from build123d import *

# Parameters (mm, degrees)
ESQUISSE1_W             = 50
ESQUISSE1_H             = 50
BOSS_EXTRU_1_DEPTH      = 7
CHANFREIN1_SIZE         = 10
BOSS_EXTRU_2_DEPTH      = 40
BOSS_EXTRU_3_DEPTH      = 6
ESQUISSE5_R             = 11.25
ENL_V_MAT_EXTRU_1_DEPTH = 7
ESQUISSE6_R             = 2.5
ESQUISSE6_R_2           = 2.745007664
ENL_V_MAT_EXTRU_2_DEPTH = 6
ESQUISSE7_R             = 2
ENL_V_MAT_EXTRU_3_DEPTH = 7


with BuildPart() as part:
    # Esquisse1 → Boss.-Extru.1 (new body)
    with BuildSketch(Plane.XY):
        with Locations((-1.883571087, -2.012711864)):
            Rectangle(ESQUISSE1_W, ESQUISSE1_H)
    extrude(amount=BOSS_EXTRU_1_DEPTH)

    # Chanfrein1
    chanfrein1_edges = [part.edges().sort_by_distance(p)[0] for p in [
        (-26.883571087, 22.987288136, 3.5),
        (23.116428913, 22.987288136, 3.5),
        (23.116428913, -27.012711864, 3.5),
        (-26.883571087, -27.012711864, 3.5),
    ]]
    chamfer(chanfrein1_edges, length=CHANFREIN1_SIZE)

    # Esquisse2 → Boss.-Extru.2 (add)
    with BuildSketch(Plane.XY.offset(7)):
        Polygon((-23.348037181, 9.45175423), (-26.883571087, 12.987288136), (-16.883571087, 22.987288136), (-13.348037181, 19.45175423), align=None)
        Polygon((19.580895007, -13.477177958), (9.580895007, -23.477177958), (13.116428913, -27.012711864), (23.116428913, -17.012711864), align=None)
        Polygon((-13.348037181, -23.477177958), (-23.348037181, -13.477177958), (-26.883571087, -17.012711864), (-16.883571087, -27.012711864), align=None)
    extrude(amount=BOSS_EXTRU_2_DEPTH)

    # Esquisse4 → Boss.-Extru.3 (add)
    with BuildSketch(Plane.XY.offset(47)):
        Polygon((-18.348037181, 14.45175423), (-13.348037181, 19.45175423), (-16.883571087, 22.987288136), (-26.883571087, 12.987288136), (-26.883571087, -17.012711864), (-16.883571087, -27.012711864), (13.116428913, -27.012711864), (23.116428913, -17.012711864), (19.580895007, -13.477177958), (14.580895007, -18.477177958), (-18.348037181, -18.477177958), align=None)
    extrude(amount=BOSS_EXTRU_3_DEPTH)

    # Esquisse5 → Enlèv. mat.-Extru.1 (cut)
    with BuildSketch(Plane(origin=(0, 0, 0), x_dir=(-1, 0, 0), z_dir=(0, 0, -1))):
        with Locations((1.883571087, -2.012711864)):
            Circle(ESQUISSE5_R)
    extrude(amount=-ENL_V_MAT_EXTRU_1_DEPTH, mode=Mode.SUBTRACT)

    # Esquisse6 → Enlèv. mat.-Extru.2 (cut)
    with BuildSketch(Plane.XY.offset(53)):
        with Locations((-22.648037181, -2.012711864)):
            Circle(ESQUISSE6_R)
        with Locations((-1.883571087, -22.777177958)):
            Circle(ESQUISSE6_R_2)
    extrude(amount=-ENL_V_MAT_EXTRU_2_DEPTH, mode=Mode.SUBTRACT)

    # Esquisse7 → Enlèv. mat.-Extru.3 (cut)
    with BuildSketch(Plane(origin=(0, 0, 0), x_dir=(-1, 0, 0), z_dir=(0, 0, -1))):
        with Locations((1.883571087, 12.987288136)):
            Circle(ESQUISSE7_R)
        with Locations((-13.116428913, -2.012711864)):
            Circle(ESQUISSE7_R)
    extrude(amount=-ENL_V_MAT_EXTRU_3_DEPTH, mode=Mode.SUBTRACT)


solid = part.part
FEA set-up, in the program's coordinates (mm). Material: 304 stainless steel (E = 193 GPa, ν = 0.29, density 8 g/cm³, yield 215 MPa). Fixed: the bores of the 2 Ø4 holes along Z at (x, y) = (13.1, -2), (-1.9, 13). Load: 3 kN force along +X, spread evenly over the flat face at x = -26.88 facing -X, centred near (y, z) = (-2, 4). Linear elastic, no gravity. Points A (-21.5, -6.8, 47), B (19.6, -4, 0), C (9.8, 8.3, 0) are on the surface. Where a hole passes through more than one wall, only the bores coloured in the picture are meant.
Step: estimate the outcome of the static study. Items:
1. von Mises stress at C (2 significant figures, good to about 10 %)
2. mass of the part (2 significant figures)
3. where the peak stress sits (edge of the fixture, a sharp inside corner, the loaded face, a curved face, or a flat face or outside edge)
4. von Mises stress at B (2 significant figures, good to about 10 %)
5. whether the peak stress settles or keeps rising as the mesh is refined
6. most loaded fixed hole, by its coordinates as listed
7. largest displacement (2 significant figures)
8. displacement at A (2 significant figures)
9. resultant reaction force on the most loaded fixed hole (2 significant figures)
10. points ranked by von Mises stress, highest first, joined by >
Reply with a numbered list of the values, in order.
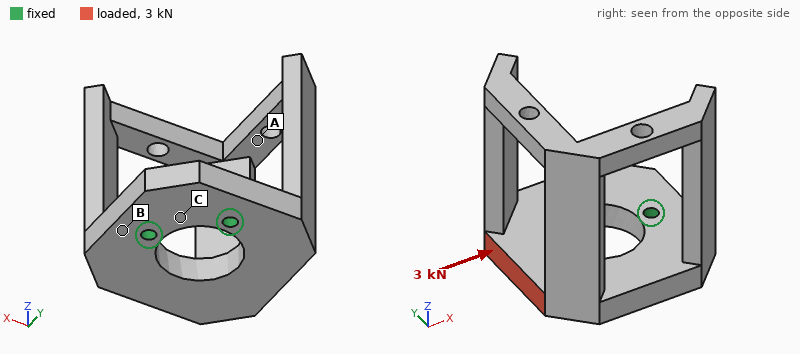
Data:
1. 13 MPa
2. 200 g
3. edge of the fixture
4. 23 MPa
5. keeps rising
6. (13.1, -2)
7. 15 µm
8. 11 µm
9. 1.8 kN
10. B > C > A
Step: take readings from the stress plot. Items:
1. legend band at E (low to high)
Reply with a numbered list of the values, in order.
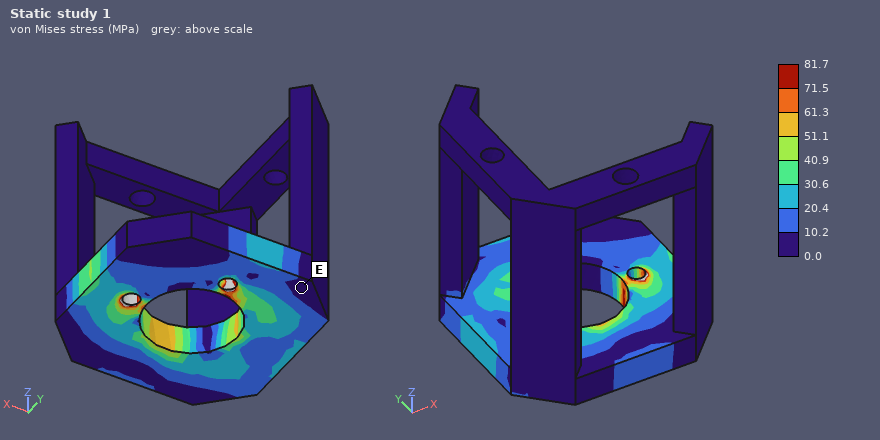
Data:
1. 0.0 to 10.2 MPa
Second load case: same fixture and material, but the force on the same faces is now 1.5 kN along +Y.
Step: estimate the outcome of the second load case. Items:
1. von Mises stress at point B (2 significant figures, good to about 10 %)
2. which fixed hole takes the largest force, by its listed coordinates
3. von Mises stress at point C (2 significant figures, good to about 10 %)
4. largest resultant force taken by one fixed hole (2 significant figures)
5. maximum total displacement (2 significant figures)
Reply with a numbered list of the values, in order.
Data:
1. 16 MPa
2. (-1.9, 13)
3. 14 MPa
4. 2.3 kN
5. 15 µm
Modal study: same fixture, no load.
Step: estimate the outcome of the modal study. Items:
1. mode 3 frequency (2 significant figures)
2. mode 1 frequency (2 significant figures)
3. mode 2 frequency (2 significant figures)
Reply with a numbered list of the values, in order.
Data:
1. 3300 Hz
2. 1300 Hz
3. 1500 Hz
